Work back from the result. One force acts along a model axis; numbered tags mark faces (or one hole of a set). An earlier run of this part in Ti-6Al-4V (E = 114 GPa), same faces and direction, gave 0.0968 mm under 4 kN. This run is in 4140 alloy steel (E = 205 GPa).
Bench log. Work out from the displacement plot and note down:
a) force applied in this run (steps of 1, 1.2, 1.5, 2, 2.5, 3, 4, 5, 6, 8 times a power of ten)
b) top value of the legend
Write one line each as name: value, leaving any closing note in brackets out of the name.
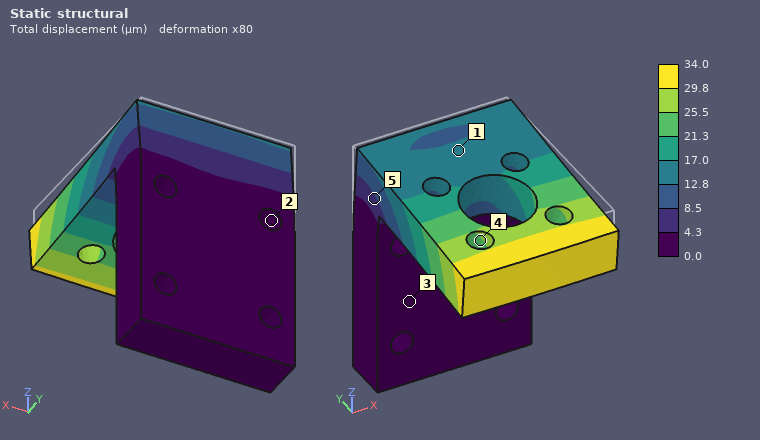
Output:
force applied in this run: 2.5 kN
top value of the legend: 34.0 µm
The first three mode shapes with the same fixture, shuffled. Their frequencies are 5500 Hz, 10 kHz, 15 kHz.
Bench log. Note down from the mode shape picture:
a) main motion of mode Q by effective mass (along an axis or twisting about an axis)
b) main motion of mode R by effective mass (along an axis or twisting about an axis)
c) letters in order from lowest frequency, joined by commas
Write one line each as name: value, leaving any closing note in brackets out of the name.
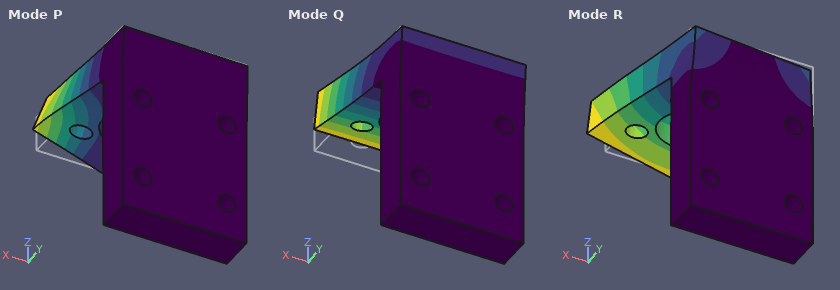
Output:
main motion of mode Q by effective mass: along Z
main motion of mode R by effective mass: along X
letters in order from lowest frequency, joined by commas: Q, R, P
